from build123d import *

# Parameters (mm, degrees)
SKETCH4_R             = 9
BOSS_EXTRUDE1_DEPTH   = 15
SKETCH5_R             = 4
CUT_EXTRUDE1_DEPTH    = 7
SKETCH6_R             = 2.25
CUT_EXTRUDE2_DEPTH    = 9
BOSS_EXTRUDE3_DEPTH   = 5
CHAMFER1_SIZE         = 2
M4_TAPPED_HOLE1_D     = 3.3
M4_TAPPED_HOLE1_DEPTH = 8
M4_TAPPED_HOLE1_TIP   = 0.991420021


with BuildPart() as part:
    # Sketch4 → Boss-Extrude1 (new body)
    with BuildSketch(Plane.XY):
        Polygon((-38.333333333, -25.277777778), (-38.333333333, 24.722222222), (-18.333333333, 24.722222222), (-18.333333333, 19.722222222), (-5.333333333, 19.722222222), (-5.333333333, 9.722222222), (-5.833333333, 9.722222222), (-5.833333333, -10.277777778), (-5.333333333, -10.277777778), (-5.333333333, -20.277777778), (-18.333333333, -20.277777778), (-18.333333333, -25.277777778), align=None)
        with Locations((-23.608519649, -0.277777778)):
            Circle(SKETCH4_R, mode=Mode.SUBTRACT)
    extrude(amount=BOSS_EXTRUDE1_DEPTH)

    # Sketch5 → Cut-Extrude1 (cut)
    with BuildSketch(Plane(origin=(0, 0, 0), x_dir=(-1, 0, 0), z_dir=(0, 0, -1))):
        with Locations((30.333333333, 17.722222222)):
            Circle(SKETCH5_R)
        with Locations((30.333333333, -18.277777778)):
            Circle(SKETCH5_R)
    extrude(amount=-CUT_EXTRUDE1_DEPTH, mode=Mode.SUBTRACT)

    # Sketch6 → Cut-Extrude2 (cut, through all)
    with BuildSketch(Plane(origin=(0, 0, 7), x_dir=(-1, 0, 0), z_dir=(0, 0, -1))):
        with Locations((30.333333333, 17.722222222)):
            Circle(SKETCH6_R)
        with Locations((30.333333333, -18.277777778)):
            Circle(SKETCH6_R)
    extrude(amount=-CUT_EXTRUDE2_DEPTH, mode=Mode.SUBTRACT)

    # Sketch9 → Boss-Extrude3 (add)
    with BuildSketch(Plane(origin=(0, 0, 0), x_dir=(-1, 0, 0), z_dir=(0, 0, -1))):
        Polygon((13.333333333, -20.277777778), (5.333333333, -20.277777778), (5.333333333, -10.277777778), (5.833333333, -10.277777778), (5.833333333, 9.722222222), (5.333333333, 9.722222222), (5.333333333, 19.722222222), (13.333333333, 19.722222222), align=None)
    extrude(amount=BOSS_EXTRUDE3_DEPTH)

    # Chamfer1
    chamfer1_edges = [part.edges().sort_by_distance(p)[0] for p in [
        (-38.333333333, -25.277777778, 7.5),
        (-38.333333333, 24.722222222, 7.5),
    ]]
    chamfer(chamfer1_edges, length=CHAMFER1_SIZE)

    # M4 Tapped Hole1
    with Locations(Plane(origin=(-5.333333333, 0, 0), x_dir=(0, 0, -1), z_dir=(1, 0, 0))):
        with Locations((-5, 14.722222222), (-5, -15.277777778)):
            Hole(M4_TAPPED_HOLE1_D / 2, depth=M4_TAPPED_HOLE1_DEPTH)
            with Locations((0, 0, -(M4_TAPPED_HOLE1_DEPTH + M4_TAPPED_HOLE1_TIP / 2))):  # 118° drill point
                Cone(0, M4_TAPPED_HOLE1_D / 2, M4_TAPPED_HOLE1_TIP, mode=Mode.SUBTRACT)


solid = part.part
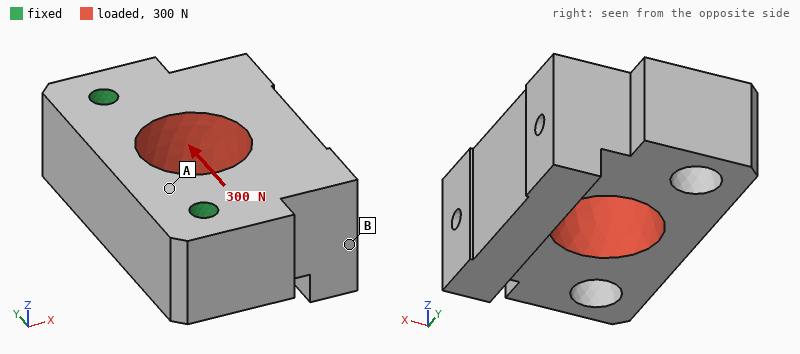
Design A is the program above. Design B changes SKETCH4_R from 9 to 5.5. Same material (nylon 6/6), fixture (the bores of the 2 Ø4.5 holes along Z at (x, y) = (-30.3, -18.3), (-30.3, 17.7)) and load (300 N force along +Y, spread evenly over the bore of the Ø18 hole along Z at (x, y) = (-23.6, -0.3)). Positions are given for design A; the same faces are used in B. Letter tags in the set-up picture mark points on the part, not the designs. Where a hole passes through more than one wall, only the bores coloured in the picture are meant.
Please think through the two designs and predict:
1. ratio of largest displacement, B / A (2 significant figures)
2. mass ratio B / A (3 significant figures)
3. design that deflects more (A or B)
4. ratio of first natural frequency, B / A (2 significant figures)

0.66
1.12
A
0.99
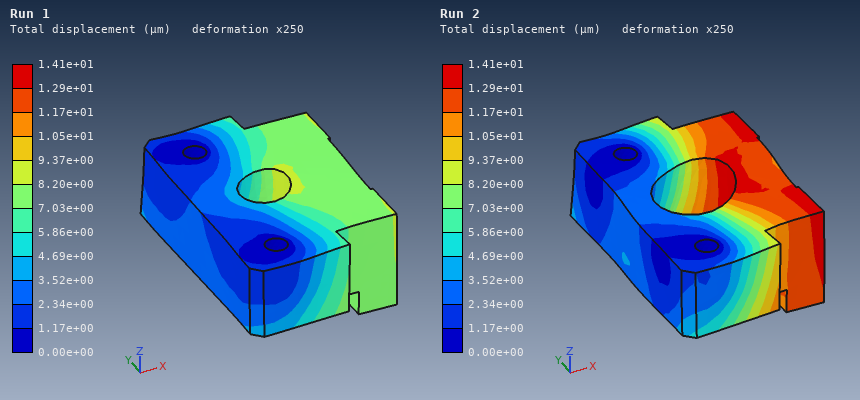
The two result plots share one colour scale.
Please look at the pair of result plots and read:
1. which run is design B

Run 1
